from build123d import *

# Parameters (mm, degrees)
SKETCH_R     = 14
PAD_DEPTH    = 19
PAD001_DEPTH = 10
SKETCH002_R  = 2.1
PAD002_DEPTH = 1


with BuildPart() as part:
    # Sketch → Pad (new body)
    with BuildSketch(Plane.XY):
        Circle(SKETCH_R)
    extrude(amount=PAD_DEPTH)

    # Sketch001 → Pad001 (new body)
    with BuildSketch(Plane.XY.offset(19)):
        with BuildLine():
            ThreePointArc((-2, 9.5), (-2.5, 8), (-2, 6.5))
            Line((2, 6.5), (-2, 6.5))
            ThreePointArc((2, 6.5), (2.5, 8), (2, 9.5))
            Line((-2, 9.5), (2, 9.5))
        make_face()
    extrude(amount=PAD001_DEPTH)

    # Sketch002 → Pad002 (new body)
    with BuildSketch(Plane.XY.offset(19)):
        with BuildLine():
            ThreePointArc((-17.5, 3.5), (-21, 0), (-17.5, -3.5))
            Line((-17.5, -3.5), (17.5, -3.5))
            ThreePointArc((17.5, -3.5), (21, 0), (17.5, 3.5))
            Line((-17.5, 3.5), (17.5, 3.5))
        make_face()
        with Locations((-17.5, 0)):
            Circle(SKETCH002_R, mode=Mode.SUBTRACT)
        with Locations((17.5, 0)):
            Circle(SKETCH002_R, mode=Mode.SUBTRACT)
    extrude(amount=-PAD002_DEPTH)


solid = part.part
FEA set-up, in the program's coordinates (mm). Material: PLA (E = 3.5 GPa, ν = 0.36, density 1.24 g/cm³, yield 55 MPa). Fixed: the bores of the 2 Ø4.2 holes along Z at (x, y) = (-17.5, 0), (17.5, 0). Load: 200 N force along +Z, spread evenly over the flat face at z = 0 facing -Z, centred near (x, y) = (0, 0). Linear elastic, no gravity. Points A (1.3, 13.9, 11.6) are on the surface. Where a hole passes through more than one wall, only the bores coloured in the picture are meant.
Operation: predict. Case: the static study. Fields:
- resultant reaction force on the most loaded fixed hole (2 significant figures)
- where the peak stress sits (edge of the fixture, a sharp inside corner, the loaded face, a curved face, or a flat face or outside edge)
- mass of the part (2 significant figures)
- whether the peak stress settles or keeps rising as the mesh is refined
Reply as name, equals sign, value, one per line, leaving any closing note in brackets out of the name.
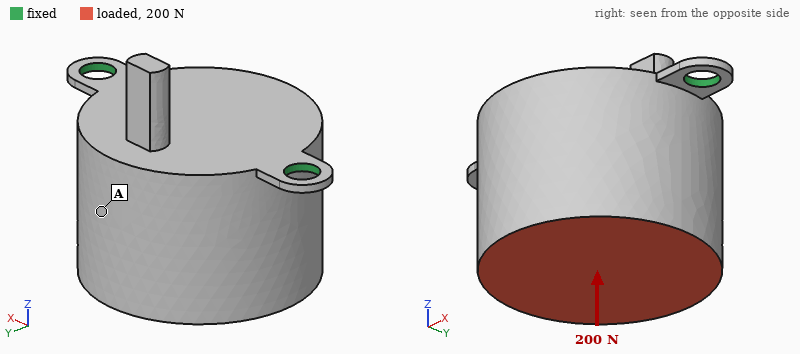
resultant reaction force on the most loaded fixed hole = 120 N
where the peak stress sits = edge of the fixture
mass of the part = 15 g
whether the peak stress settles or keeps rising as the mesh is refined = keeps rising
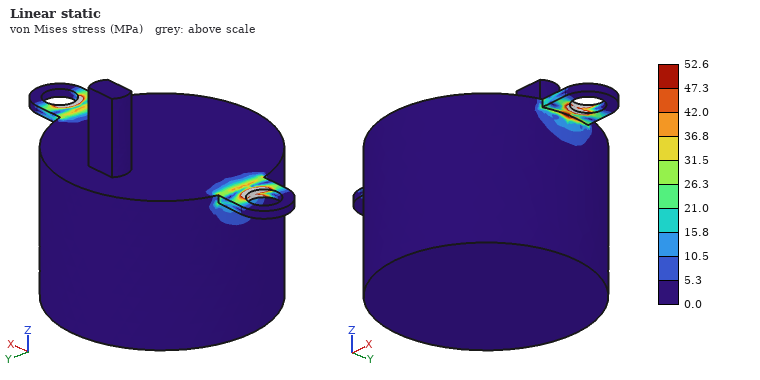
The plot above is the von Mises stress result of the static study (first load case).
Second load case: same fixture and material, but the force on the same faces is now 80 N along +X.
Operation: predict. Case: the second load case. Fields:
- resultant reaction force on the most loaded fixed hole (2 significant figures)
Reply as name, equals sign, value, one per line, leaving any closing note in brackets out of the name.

resultant reaction force on the most loaded fixed hole = 64 N
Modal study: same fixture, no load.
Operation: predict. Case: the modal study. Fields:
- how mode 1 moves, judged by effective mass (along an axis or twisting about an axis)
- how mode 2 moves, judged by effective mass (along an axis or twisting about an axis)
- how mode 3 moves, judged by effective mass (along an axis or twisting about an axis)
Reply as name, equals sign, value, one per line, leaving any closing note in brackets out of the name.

how mode 1 moves, judged by effective mass = along Y
how mode 2 moves, judged by effective mass = along Z
how mode 3 moves, judged by effective mass = along X
